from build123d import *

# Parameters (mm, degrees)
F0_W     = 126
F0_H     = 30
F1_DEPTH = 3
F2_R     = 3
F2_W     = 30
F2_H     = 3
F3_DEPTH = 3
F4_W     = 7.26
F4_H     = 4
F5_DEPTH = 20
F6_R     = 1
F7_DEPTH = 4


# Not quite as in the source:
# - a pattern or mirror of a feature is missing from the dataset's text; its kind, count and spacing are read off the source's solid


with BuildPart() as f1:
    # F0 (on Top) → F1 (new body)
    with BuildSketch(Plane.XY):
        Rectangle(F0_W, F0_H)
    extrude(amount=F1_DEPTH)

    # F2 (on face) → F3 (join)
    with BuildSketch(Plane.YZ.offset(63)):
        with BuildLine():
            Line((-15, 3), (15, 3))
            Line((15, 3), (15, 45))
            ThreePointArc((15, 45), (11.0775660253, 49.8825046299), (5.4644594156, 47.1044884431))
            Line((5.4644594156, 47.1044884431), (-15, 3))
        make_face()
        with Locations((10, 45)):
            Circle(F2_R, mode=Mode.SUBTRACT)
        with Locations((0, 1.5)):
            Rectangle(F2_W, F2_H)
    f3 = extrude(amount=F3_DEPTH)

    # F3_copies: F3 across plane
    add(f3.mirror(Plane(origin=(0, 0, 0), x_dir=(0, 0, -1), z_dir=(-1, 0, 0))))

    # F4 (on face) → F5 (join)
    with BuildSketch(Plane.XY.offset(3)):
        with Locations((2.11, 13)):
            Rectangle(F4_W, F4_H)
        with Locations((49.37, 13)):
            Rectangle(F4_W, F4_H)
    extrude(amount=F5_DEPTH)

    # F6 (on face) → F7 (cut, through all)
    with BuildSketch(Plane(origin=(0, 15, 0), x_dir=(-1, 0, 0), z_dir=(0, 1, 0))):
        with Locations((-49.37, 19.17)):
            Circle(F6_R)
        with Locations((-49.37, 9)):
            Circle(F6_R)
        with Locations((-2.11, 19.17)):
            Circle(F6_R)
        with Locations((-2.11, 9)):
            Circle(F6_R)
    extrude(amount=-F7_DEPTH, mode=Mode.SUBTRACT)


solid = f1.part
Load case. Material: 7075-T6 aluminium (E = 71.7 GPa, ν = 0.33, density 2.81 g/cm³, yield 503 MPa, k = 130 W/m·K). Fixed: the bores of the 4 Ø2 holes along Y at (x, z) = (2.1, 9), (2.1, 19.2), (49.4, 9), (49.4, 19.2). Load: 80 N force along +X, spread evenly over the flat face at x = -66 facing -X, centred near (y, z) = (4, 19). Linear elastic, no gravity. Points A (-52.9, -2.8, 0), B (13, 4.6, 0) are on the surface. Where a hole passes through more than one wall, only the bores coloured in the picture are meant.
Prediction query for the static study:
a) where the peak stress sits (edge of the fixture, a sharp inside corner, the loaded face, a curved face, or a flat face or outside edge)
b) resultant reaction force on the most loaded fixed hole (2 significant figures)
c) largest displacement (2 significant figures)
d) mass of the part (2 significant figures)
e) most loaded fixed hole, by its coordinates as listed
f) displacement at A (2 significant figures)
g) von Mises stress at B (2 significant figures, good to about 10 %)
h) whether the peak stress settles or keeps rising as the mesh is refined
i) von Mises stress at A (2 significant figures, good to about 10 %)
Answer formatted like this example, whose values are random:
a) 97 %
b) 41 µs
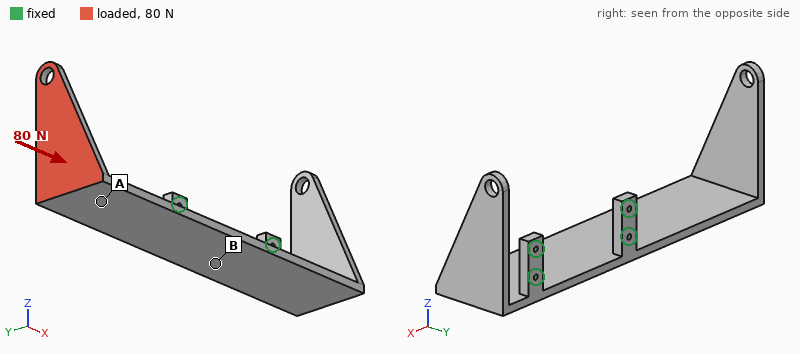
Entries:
a) a sharp inside corner
b) 93 N
c) 1.4 mm
d) 51 g
e) (2.1, 9)
f) 0.52 mm
g) 7.6 MPa
h) keeps rising
i) 26 MPa
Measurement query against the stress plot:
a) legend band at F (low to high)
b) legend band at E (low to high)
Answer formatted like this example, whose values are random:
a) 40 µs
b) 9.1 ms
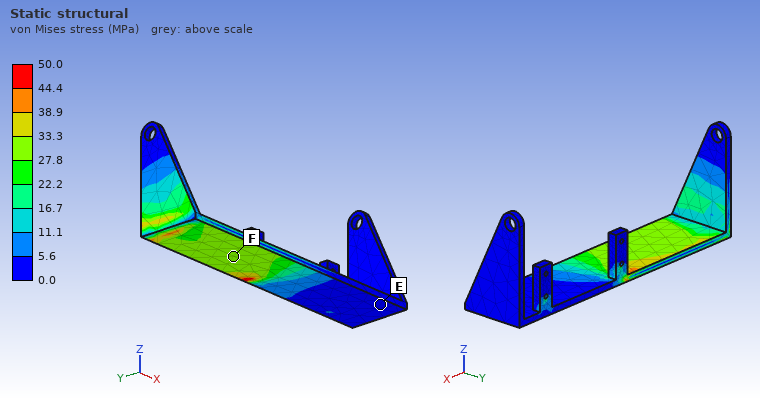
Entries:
a) 27.8 to 33.3 MPa
b) 0.0 to 5.6 MPa
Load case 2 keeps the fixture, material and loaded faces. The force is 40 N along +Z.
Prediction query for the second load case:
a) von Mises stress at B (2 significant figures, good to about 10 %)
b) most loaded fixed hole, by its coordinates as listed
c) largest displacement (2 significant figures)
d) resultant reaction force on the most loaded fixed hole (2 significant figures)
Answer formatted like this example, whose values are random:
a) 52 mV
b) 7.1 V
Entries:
a) 17 MPa
b) (49.4, 9)
c) 1.5 mm
d) 130 N
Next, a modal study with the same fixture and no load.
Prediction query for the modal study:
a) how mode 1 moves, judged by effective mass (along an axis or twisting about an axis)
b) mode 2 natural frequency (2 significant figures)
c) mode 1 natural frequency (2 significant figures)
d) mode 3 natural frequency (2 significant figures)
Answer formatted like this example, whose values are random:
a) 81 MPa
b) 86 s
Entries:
a) along Z
b) 650 Hz
c) 270 Hz
d) 950 Hz
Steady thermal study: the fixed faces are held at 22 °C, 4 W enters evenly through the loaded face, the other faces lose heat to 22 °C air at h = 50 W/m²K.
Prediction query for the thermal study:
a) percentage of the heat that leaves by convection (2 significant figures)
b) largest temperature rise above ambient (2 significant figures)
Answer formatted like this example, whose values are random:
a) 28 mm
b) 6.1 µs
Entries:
a) 72 %
b) 19 K
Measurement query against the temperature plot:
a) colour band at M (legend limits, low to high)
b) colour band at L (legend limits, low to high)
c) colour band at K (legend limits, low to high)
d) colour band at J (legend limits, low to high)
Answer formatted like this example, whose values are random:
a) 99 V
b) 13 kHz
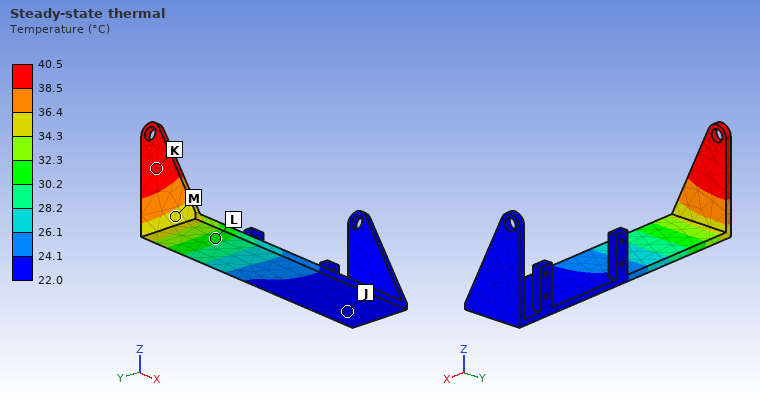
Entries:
a) 34.3 to 36.4 °C
b) 30.2 to 32.3 °C
c) 38.5 to 40.5 °C
d) 22.0 to 24.1 °C
